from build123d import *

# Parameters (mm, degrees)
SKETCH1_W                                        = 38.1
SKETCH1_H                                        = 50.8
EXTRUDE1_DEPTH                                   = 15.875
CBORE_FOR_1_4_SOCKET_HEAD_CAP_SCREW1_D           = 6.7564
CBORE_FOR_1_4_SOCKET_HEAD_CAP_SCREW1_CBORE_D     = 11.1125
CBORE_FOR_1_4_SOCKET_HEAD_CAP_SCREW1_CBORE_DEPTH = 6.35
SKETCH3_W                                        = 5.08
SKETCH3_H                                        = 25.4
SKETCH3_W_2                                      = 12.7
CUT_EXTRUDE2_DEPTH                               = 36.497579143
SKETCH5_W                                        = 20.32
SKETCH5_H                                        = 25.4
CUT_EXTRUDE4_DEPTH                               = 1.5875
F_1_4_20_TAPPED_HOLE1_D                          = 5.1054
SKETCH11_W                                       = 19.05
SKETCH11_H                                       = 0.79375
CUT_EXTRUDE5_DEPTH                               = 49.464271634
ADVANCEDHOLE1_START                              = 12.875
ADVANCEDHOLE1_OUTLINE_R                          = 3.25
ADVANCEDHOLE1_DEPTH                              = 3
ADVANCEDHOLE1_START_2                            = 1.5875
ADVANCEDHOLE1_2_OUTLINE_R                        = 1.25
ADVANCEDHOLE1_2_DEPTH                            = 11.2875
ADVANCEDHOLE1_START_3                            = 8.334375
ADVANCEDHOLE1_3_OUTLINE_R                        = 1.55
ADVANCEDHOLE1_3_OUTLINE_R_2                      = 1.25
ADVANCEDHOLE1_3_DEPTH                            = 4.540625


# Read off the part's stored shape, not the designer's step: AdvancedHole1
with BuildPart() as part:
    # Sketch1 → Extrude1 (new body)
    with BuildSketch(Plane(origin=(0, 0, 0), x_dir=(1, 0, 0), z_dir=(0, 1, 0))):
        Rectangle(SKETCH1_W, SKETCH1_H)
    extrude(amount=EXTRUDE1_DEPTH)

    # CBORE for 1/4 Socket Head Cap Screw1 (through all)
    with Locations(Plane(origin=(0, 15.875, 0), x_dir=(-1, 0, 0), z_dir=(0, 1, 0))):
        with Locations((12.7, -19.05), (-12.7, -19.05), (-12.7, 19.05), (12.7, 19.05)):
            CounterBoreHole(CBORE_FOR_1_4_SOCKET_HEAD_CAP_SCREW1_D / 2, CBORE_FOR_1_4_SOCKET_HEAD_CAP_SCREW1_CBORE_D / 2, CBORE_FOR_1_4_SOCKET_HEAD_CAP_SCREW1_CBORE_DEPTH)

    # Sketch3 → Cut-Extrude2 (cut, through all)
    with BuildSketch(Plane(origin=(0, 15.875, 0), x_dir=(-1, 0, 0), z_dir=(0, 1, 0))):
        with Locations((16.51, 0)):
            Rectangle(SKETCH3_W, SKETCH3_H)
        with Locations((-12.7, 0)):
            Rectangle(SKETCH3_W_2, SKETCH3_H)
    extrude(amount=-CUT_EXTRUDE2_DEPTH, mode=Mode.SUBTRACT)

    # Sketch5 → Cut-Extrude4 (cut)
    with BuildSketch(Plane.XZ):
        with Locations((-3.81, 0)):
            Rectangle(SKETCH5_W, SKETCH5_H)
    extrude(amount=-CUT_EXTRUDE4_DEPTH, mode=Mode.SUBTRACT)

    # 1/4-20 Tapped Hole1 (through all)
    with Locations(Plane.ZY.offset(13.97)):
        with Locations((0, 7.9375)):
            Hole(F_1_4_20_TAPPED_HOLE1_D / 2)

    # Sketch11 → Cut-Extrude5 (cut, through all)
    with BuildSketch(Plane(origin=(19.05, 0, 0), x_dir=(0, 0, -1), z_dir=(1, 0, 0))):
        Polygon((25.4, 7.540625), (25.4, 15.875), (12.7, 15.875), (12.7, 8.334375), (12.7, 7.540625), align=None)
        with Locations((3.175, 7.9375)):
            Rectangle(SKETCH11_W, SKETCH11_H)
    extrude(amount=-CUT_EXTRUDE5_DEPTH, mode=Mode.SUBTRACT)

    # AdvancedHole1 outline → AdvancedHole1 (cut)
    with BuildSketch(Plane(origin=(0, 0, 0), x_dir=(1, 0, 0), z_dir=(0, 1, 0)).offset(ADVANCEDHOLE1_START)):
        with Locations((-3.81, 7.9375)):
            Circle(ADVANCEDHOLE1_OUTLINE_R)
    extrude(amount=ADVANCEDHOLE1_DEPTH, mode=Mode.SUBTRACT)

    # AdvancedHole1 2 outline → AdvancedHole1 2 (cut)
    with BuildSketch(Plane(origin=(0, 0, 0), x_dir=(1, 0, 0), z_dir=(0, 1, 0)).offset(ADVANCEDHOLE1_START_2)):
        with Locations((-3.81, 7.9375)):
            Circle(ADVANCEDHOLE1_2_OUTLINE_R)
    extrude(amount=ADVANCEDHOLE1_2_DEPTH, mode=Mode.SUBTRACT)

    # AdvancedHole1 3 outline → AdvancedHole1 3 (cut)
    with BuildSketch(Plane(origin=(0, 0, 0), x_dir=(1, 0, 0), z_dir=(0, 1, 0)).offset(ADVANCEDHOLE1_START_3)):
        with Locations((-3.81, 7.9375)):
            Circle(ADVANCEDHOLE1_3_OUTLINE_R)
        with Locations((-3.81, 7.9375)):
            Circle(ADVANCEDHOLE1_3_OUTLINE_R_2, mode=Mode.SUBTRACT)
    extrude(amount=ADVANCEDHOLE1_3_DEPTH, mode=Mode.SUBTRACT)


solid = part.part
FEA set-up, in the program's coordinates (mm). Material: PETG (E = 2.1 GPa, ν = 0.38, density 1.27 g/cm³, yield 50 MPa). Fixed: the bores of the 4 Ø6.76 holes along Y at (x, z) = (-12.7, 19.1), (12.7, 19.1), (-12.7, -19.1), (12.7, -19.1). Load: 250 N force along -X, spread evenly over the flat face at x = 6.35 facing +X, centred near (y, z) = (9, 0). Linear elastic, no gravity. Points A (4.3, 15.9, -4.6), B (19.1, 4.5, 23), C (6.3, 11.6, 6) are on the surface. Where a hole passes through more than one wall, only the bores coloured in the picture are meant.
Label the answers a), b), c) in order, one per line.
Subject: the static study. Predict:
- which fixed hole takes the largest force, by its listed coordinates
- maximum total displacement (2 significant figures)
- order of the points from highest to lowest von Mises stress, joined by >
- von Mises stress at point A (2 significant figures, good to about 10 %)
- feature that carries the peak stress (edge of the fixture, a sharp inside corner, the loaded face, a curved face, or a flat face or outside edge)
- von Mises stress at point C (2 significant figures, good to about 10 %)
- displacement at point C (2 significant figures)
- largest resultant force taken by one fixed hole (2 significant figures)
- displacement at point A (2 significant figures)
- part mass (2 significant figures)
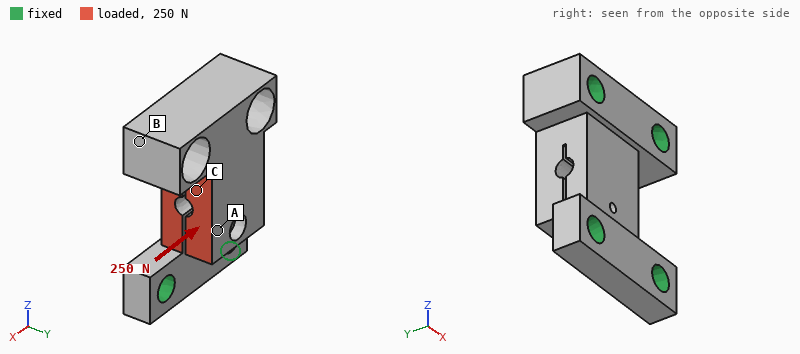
a) (-12.7, 19.1)
b) 84 µm
c) C > A > B
d) 1.0 MPa
e) the loaded face
f) 2.2 MPa
g) 30 µm
h) 150 N
i) 55 µm
j) 20 g
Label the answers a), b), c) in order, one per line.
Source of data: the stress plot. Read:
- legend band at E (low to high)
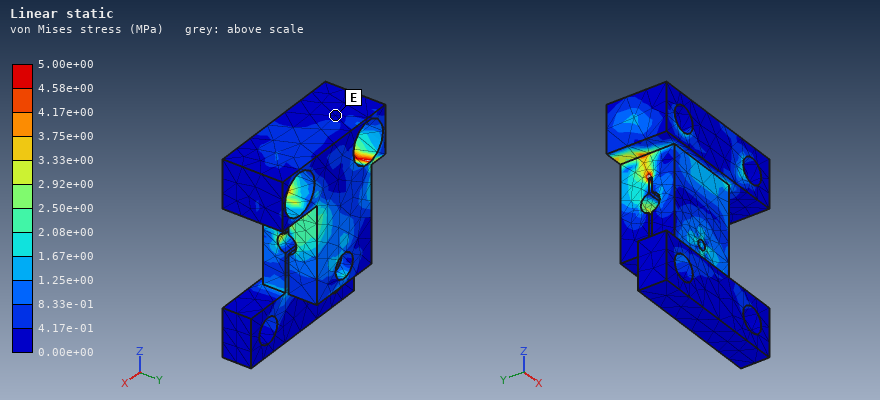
a) 0.00e+00 to 4.17e-01 MPa
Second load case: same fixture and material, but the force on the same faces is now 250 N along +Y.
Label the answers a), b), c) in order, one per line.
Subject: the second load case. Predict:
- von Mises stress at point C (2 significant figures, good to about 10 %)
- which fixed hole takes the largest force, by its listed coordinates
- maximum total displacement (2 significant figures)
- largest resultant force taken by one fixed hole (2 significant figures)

a) 5.6 MPa
b) (12.7, 19.1)
c) 0.42 mm
d) 140 N
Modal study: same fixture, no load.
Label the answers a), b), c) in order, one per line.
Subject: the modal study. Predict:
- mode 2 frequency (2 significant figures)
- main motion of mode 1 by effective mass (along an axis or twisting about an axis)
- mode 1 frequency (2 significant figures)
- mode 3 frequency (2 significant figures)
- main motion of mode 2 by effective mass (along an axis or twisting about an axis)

a) 3900 Hz
b) along Y
c) 2100 Hz
d) 5100 Hz
e) along X
